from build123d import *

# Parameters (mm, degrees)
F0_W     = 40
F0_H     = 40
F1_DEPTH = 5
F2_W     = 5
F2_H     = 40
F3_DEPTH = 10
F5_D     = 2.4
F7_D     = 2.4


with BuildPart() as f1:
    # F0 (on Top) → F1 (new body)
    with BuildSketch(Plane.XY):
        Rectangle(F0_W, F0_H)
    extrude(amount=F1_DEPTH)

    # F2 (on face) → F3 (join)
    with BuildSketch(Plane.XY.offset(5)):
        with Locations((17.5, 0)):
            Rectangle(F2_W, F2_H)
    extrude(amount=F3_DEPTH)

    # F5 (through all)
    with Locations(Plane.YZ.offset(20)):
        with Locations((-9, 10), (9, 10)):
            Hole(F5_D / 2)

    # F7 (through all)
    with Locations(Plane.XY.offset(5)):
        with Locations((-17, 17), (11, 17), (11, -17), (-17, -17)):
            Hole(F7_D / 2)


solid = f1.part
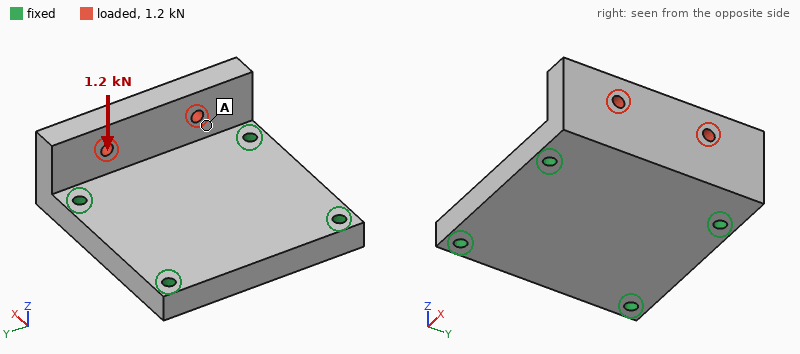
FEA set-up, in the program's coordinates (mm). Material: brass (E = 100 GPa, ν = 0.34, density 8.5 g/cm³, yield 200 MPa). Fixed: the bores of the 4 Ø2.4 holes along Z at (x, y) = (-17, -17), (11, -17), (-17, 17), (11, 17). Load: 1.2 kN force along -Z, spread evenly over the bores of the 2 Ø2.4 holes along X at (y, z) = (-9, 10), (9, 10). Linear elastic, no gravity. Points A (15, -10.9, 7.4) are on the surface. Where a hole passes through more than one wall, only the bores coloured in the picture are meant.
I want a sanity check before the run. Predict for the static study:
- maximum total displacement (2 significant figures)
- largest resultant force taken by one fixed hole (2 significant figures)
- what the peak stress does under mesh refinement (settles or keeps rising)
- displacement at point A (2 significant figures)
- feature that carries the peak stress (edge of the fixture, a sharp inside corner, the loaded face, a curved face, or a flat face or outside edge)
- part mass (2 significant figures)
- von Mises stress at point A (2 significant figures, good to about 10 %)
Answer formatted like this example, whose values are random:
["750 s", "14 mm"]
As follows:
["19 µm", "670 N", "keeps rising", "8.4 µm", "edge of the fixture", "84 g", "19 MPa"]
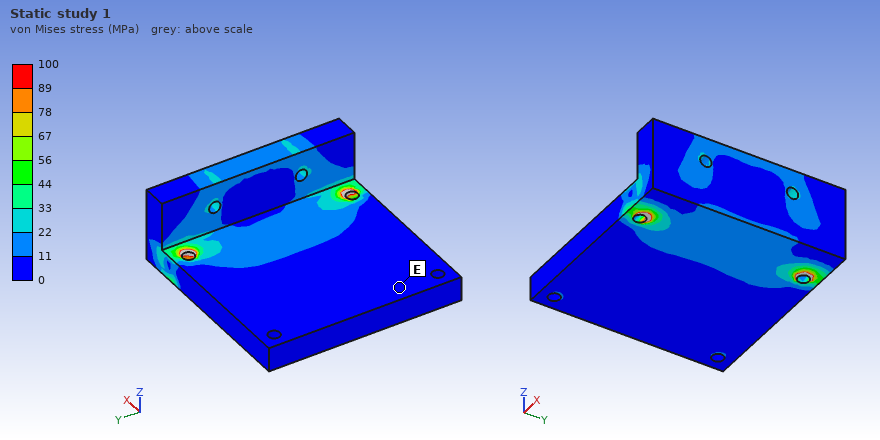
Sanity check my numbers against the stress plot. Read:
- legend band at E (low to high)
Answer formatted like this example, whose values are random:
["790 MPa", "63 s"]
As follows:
["0 to 11 MPa"]
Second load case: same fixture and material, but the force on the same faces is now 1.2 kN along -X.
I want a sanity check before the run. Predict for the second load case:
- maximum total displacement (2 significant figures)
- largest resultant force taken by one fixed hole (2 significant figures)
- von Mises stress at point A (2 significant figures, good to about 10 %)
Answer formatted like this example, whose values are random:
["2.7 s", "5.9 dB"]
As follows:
["33 µm", "420 N", "26 MPa"]
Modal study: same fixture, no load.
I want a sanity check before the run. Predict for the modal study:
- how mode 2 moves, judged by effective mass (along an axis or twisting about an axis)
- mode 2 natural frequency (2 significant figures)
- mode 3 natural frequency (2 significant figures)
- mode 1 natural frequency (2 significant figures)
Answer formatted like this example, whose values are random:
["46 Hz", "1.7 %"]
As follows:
["along Z", "11 kHz", "13 kHz", "7900 Hz"]
